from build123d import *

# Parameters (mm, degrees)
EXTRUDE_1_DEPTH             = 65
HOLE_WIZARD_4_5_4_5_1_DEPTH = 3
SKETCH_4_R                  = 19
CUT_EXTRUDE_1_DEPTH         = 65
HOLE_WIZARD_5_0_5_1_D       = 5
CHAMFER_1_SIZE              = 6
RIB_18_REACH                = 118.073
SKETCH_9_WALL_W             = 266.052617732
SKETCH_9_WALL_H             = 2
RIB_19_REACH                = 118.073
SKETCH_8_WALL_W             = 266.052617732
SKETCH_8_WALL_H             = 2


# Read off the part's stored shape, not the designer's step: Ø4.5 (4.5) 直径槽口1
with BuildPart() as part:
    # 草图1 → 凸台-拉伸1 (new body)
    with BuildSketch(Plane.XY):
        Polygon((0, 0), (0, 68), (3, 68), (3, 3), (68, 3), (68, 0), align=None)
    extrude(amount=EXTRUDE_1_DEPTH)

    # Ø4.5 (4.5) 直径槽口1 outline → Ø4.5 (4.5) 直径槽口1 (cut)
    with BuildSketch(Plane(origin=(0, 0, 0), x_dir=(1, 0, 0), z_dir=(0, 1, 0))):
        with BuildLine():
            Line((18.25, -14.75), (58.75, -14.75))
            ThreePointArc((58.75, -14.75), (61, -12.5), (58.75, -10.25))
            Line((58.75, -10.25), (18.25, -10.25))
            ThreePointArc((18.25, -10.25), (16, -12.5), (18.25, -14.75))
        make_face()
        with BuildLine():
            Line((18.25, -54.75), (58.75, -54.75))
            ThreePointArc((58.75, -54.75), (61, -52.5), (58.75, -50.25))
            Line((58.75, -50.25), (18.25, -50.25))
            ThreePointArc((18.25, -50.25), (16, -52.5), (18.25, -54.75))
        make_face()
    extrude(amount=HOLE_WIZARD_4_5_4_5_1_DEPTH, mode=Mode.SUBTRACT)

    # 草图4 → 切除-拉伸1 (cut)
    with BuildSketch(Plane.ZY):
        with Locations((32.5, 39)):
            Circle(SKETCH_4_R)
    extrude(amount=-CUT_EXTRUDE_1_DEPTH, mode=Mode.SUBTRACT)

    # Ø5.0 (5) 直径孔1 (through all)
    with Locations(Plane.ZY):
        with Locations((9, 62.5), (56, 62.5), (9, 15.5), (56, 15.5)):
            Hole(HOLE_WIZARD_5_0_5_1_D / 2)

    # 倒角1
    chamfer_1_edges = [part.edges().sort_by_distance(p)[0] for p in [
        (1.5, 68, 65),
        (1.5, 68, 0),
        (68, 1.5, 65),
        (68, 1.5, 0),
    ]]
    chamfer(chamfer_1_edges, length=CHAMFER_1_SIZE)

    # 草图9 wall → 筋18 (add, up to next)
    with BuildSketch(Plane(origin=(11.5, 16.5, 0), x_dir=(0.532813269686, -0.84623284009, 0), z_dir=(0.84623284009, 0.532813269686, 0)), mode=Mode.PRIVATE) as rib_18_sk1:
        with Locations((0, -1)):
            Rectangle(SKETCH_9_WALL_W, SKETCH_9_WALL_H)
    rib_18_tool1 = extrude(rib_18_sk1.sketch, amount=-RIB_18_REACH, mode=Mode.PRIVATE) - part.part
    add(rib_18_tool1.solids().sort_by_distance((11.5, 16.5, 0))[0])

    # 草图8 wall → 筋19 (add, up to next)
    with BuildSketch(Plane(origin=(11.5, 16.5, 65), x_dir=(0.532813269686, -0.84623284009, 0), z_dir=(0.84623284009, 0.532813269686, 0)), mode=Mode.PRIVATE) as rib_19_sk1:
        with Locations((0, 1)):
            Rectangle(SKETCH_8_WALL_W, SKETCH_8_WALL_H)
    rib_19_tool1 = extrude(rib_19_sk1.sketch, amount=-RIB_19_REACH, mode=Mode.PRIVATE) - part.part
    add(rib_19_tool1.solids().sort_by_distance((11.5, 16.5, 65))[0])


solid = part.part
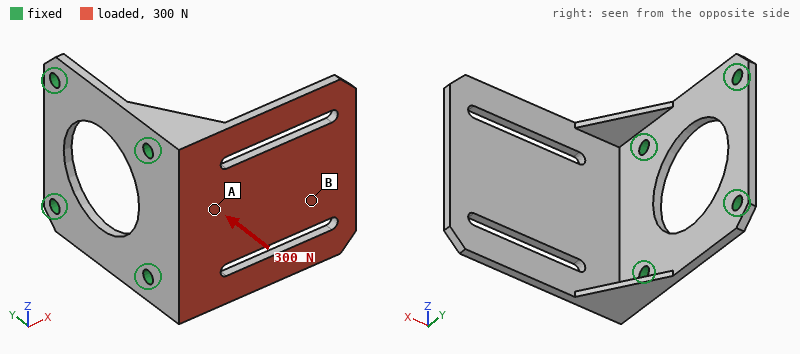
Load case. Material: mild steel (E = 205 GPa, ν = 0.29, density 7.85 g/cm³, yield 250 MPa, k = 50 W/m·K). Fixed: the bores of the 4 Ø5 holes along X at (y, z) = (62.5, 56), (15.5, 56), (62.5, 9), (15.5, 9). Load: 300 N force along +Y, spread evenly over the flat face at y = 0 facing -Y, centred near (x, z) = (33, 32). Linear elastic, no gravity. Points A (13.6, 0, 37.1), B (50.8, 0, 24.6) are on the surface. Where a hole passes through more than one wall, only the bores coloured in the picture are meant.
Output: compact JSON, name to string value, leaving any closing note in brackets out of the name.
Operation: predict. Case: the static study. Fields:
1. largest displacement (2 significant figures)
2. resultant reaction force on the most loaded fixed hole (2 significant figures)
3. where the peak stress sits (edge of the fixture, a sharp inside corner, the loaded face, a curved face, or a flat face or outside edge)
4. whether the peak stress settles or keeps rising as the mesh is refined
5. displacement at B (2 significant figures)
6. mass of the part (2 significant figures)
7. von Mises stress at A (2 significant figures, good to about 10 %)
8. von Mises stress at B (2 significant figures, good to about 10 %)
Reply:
{"largest displacement": "0.35 mm", "resultant reaction force on the most loaded fixed hole": "150 N", "where the peak stress sits": "edge of the fixture", "whether the peak stress settles or keeps rising as the mesh is refined": "keeps rising", "displacement at B": "0.23 mm", "mass of the part": "170 g", "von Mises stress at A": "39 MPa", "von Mises stress at B": "13 MPa"}
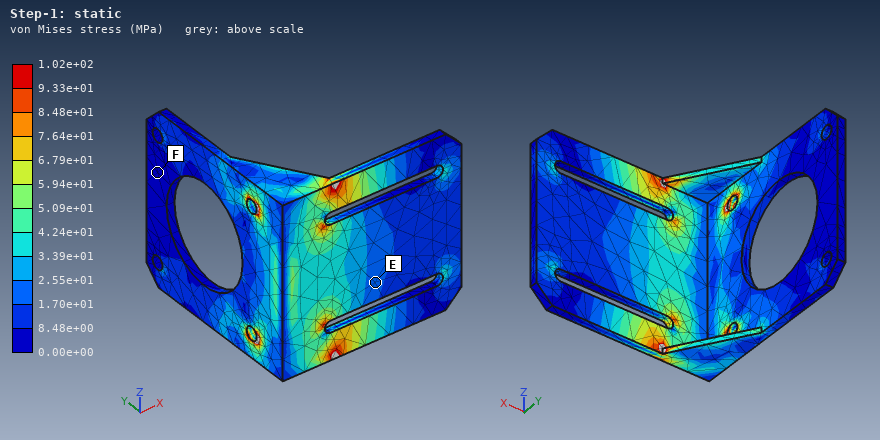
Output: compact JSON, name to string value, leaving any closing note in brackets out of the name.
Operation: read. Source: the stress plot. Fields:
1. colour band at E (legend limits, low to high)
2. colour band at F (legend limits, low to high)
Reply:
{"colour band at E": "1.70e+01 to 2.55e+01 MPa", "colour band at F": "0.00e+00 to 8.48e+00 MPa"}
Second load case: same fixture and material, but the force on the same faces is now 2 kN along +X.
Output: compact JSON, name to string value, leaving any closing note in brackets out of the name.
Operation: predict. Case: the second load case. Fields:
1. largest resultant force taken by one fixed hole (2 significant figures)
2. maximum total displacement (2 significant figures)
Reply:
{"largest resultant force taken by one fixed hole": "1.1 kN", "maximum total displacement": "0.36 mm"}
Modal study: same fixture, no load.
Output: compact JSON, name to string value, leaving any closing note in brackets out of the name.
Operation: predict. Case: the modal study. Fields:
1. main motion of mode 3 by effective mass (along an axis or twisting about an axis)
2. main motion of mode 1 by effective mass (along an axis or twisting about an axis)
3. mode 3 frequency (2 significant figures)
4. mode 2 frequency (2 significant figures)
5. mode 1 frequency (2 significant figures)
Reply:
{"main motion of mode 3 by effective mass": "along Z", "main motion of mode 1 by effective mass": "along Y", "mode 3 frequency": "2500 Hz", "mode 2 frequency": "1600 Hz", "mode 1 frequency": "600 Hz"}
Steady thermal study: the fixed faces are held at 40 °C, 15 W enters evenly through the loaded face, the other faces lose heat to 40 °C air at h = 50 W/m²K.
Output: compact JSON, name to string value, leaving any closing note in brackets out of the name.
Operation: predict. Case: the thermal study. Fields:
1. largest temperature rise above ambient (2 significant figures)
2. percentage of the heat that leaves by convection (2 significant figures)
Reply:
{"largest temperature rise above ambient": "35 K", "percentage of the heat that leaves by convection": "54 %"}
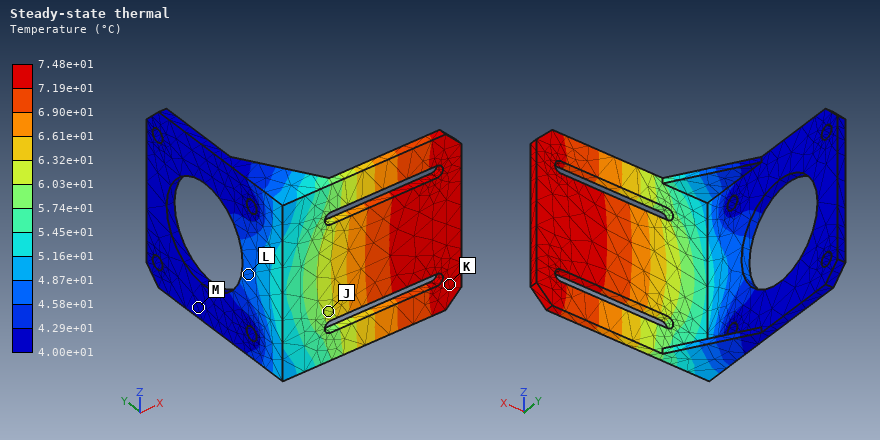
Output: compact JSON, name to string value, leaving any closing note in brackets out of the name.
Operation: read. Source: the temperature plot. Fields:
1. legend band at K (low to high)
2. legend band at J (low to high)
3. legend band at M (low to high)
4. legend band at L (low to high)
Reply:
{"legend band at K": "7.19e+01 to 7.48e+01 °C", "legend band at J": "6.03e+01 to 6.32e+01 °C", "legend band at M": "4.00e+01 to 4.29e+01 °C", "legend band at L": "4.58e+01 to 4.87e+01 °C"}
